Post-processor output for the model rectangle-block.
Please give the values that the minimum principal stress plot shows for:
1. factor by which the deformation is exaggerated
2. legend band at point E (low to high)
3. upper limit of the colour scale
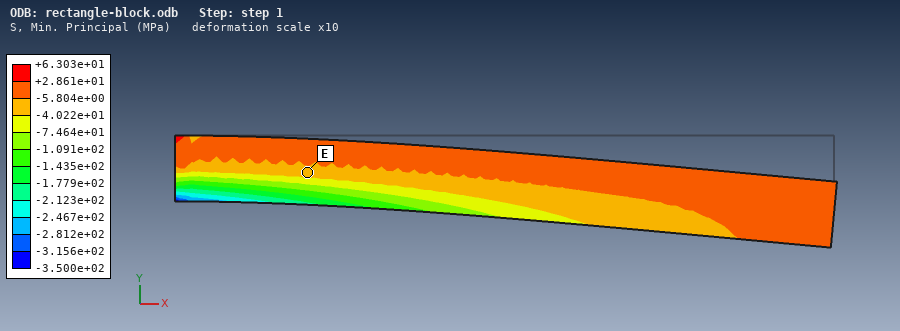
10
-4.022e+01 to -5.804e+00 MPa
+6.303e+01 MPa
